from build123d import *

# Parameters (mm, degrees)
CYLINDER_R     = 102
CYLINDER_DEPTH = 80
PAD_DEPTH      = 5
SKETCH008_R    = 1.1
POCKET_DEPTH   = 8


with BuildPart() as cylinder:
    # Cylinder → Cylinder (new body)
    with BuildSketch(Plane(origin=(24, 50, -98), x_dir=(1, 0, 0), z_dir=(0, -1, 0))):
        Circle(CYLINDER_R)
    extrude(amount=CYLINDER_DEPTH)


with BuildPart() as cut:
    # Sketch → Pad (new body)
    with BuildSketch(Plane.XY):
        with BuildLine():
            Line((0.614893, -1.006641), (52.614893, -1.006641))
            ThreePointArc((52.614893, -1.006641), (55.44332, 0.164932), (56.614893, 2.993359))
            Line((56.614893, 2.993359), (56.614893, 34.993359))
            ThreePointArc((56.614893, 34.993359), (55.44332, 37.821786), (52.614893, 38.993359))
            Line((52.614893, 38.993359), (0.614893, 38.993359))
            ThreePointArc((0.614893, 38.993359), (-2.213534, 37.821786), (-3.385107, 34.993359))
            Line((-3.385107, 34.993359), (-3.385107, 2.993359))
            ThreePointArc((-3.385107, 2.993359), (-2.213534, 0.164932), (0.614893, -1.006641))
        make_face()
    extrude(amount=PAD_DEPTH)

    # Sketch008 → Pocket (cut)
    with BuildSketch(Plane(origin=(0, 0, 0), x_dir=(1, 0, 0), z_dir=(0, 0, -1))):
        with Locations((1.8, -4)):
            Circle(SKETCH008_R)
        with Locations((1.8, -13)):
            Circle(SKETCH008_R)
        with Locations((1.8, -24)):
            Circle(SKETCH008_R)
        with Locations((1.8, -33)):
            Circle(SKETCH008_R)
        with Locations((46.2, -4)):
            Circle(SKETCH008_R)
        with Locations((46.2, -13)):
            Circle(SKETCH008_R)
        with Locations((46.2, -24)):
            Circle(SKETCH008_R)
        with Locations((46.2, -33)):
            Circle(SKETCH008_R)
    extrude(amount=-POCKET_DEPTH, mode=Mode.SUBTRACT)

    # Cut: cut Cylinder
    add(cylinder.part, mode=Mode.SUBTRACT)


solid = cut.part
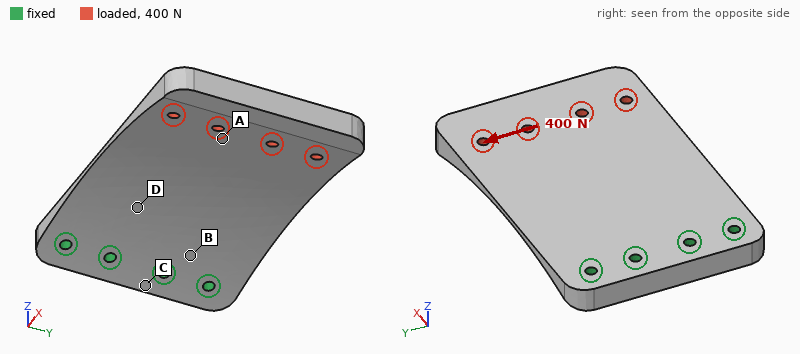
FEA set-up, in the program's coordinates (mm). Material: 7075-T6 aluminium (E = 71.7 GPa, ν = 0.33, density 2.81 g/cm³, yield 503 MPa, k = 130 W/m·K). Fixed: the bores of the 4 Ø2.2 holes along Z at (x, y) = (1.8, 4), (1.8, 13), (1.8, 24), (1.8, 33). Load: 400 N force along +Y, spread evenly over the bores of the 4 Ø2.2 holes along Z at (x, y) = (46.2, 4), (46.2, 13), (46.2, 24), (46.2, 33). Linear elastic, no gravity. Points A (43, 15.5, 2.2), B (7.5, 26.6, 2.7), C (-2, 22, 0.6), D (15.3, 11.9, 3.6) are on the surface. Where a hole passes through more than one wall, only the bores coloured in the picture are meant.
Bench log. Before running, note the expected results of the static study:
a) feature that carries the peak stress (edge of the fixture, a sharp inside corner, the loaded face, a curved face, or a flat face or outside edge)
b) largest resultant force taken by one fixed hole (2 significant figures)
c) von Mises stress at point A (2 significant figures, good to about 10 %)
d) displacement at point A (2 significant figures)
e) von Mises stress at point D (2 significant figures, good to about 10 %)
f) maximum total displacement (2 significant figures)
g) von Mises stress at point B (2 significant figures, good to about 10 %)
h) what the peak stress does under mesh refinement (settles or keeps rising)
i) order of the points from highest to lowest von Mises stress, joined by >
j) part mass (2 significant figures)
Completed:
edge of the fixture
570 N
11 MPa
0.063 mm
39 MPa
0.21 mm
23 MPa
keeps rising
D > B > A > C
16 g
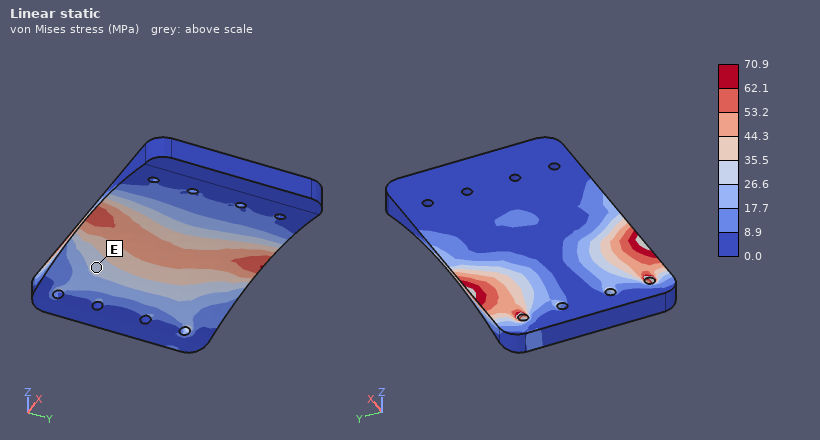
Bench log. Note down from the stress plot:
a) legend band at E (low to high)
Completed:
26.6 to 35.5 MPa
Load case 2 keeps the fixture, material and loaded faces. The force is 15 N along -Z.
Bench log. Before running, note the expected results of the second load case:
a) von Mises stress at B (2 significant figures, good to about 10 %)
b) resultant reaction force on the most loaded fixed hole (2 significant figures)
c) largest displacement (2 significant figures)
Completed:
15 MPa
9.6 N
0.75 mm
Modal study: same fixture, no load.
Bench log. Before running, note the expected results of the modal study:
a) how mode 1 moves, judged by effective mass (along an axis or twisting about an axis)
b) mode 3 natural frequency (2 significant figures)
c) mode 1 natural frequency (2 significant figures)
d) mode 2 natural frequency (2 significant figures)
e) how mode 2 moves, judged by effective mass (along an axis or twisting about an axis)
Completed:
along Z
2900 Hz
270 Hz
1100 Hz
twisting about X
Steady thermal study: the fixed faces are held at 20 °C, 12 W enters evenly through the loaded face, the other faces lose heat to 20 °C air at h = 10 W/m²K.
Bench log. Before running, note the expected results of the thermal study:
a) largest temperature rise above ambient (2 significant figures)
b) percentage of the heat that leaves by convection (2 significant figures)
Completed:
60 K
14 %
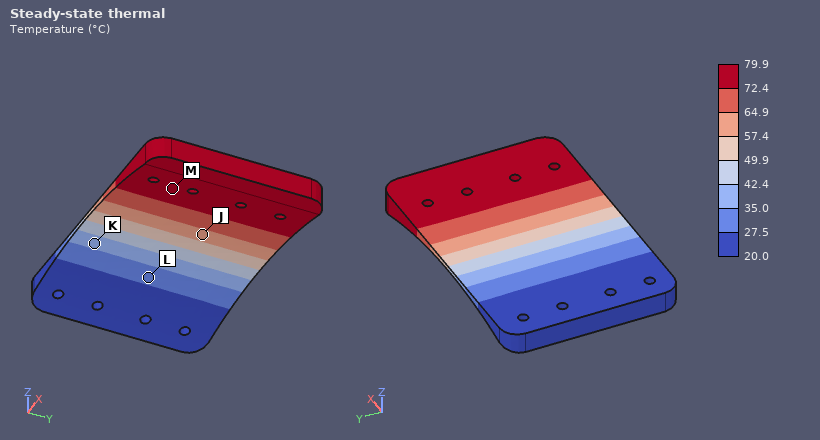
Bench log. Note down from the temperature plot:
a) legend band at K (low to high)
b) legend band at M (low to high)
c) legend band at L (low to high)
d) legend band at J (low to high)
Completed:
35.0 to 42.4 °C
72.4 to 79.9 °C
27.5 to 35.0 °C
57.4 to 64.9 °C
